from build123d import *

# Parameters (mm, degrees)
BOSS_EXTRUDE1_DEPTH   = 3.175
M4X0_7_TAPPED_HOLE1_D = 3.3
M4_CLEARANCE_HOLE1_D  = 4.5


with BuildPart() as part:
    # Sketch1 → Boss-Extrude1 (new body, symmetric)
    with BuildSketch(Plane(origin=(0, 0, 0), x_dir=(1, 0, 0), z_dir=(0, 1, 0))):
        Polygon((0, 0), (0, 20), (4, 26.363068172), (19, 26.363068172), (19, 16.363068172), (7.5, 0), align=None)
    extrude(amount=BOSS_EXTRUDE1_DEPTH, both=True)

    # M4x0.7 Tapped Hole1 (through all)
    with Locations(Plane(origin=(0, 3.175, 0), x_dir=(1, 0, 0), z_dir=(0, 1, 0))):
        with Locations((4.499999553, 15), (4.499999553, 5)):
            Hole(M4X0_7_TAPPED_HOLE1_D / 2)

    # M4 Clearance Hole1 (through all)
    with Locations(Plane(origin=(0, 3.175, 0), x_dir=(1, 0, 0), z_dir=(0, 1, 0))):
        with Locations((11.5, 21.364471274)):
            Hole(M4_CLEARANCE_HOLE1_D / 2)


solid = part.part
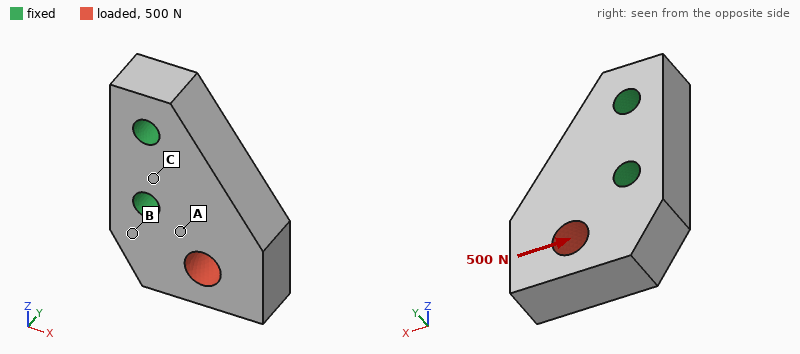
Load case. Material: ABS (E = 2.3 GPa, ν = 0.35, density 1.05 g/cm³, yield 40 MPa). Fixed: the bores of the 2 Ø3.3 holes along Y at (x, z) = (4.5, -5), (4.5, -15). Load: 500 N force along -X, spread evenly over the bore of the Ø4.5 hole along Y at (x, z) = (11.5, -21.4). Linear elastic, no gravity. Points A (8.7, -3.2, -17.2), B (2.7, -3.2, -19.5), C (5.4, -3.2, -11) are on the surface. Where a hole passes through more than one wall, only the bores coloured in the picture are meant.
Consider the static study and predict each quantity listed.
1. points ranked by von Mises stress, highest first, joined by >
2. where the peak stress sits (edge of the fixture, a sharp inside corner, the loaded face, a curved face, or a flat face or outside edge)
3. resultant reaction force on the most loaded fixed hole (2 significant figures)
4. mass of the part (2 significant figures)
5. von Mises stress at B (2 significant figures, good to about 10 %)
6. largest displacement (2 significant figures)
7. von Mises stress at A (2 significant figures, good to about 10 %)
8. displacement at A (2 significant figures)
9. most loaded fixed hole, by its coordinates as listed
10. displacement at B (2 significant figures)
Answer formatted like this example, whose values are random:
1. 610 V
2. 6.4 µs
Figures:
1. A > B > C
2. edge of the fixture
3. 690 N
4. 2.4 g
5. 8.2 MPa
6. 0.18 mm
7. 16 MPa
8. 0.042 mm
9. (4.5, -15)
10. 0.052 mm
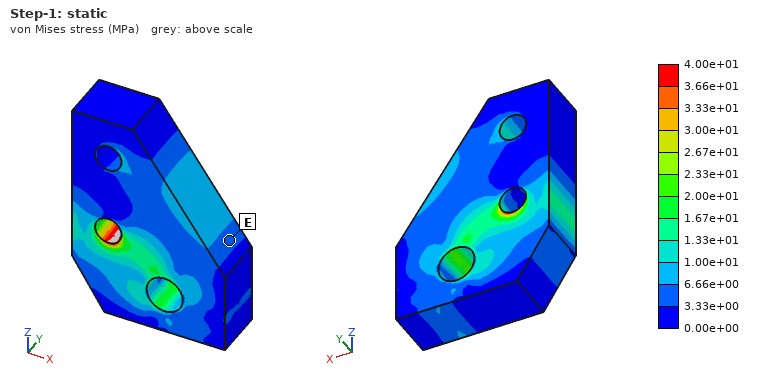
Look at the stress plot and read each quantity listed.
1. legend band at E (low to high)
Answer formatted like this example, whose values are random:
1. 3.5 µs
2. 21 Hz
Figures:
1. 3.33e+00 to 6.66e+00 MPa
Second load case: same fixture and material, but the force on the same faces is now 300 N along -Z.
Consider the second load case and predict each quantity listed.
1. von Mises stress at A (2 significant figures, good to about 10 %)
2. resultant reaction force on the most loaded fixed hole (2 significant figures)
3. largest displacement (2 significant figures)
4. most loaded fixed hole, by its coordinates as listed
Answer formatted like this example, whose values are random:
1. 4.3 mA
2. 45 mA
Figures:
1. 5.9 MPa
2. 240 N
3. 75 µm
4. (4.5, -15)
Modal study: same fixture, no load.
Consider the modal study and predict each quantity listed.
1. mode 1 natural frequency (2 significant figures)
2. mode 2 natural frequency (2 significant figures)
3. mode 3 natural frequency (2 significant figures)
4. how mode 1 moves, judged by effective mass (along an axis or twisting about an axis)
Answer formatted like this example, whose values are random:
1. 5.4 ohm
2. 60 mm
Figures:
1. 5800 Hz
2. 8600 Hz
3. 11 kHz
4. along Y
